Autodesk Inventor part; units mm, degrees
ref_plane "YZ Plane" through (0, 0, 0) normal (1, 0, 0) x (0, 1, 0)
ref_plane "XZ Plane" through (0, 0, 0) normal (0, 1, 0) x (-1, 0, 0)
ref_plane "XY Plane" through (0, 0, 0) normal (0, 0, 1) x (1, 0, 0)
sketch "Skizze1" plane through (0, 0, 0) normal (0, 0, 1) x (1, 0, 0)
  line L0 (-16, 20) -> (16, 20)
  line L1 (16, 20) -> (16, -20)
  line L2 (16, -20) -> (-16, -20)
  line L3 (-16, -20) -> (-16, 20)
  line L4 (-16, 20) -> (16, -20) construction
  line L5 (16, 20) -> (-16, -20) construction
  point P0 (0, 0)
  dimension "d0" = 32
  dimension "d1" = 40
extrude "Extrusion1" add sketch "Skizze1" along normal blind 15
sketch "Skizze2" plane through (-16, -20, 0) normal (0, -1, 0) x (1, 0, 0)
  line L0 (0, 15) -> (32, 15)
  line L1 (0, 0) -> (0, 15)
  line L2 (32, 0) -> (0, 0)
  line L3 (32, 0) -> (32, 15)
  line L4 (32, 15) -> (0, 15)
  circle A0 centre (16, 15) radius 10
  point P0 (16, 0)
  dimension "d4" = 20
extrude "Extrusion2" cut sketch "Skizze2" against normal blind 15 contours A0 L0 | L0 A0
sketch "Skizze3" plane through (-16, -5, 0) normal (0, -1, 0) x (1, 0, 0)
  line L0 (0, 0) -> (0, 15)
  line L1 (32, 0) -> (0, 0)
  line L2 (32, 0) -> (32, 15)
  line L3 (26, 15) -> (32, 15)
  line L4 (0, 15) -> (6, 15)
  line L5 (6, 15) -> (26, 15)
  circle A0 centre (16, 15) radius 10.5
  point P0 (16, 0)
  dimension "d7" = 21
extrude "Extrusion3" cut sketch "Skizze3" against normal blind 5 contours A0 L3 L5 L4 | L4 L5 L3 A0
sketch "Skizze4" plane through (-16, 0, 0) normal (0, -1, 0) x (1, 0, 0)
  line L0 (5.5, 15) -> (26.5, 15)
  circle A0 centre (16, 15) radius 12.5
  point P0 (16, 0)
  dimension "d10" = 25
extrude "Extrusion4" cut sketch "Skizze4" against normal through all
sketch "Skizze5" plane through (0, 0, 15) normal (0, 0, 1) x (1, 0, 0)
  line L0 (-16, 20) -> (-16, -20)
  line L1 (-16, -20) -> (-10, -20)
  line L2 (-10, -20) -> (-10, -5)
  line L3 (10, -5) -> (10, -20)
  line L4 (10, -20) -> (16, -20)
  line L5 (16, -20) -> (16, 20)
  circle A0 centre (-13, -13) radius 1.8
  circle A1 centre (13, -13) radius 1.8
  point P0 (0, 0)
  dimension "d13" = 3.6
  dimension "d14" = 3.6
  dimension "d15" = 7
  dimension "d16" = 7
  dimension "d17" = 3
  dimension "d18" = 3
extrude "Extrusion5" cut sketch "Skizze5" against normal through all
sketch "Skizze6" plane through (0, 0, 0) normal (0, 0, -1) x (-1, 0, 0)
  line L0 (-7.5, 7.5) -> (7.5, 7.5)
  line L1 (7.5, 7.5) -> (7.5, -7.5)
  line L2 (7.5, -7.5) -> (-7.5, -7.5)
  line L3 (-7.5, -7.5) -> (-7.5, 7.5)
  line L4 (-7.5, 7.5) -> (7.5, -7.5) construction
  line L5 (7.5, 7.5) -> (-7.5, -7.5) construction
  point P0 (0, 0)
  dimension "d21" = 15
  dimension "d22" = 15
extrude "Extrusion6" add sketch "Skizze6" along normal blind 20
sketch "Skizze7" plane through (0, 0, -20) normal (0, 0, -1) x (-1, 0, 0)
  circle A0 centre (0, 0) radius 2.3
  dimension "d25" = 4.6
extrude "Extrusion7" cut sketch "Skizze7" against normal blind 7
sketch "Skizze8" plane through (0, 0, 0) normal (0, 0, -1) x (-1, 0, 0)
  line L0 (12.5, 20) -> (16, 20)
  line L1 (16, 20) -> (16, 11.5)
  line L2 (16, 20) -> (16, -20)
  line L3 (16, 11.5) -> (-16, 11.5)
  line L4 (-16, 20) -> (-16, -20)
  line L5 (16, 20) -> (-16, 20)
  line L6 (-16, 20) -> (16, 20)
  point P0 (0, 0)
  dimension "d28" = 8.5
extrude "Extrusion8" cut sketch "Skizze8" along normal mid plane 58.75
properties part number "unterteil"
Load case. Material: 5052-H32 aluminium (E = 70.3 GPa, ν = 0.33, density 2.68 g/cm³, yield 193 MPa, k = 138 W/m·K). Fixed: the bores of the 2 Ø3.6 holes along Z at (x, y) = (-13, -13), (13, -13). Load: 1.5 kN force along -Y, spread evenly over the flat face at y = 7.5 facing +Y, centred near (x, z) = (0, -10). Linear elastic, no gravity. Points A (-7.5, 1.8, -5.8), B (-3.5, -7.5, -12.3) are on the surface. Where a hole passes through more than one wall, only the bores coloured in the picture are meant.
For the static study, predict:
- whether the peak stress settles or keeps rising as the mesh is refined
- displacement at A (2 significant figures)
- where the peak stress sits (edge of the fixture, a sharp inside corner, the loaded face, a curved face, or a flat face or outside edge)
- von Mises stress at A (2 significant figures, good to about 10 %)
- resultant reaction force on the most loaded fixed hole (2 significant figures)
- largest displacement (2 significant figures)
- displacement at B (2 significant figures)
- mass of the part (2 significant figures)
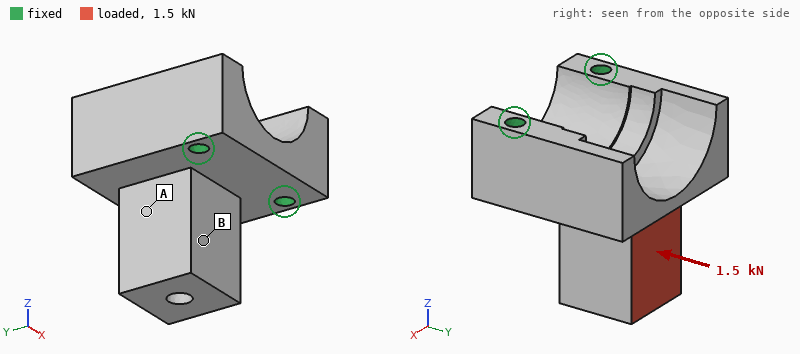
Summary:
keeps rising
23 µm
edge of the fixture
16 MPa
840 N
54 µm
32 µm
35 g
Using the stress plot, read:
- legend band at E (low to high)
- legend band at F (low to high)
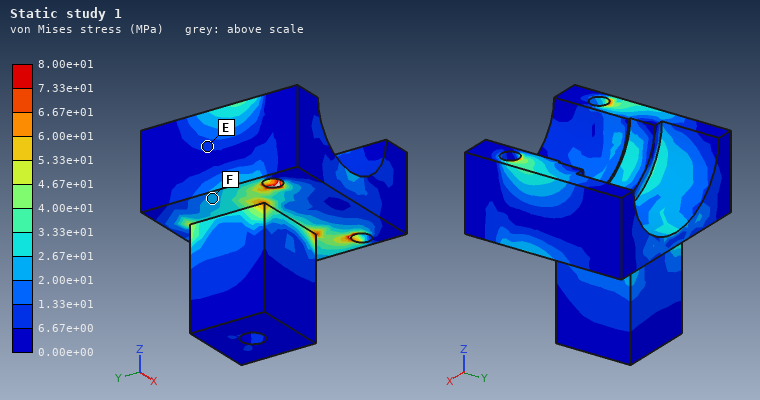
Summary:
6.67e+00 to 1.33e+01 MPa
2.00e+01 to 2.67e+01 MPa
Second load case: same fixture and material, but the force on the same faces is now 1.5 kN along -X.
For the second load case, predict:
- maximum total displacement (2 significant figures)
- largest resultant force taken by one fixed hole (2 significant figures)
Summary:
33 µm
1.7 kN
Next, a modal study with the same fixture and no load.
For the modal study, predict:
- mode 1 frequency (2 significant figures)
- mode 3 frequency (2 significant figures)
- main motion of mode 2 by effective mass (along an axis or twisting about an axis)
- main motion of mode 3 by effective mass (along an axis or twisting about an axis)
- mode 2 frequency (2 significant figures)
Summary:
8400 Hz
18 kHz
along X
along X
12 kHz
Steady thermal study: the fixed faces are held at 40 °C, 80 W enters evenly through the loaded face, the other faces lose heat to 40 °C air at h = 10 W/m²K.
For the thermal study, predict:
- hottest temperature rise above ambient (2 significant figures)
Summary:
69 K
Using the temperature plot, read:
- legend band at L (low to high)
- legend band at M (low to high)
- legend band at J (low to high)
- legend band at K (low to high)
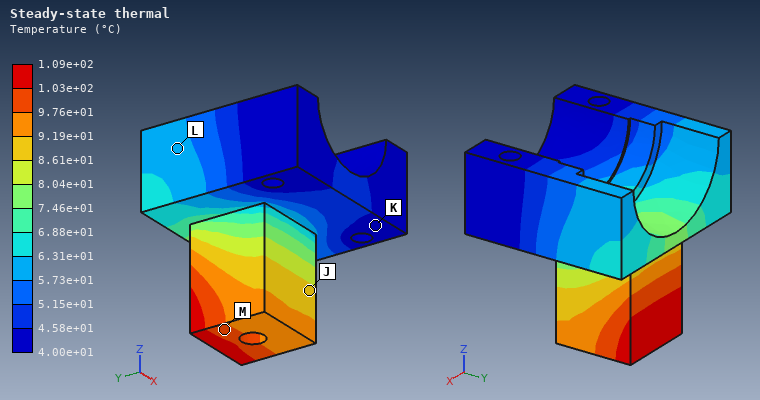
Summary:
5.73e+01 to 6.31e+01 °C
9.76e+01 to 1.03e+02 °C
8.61e+01 to 9.19e+01 °C
4.00e+01 to 4.58e+01 °C
